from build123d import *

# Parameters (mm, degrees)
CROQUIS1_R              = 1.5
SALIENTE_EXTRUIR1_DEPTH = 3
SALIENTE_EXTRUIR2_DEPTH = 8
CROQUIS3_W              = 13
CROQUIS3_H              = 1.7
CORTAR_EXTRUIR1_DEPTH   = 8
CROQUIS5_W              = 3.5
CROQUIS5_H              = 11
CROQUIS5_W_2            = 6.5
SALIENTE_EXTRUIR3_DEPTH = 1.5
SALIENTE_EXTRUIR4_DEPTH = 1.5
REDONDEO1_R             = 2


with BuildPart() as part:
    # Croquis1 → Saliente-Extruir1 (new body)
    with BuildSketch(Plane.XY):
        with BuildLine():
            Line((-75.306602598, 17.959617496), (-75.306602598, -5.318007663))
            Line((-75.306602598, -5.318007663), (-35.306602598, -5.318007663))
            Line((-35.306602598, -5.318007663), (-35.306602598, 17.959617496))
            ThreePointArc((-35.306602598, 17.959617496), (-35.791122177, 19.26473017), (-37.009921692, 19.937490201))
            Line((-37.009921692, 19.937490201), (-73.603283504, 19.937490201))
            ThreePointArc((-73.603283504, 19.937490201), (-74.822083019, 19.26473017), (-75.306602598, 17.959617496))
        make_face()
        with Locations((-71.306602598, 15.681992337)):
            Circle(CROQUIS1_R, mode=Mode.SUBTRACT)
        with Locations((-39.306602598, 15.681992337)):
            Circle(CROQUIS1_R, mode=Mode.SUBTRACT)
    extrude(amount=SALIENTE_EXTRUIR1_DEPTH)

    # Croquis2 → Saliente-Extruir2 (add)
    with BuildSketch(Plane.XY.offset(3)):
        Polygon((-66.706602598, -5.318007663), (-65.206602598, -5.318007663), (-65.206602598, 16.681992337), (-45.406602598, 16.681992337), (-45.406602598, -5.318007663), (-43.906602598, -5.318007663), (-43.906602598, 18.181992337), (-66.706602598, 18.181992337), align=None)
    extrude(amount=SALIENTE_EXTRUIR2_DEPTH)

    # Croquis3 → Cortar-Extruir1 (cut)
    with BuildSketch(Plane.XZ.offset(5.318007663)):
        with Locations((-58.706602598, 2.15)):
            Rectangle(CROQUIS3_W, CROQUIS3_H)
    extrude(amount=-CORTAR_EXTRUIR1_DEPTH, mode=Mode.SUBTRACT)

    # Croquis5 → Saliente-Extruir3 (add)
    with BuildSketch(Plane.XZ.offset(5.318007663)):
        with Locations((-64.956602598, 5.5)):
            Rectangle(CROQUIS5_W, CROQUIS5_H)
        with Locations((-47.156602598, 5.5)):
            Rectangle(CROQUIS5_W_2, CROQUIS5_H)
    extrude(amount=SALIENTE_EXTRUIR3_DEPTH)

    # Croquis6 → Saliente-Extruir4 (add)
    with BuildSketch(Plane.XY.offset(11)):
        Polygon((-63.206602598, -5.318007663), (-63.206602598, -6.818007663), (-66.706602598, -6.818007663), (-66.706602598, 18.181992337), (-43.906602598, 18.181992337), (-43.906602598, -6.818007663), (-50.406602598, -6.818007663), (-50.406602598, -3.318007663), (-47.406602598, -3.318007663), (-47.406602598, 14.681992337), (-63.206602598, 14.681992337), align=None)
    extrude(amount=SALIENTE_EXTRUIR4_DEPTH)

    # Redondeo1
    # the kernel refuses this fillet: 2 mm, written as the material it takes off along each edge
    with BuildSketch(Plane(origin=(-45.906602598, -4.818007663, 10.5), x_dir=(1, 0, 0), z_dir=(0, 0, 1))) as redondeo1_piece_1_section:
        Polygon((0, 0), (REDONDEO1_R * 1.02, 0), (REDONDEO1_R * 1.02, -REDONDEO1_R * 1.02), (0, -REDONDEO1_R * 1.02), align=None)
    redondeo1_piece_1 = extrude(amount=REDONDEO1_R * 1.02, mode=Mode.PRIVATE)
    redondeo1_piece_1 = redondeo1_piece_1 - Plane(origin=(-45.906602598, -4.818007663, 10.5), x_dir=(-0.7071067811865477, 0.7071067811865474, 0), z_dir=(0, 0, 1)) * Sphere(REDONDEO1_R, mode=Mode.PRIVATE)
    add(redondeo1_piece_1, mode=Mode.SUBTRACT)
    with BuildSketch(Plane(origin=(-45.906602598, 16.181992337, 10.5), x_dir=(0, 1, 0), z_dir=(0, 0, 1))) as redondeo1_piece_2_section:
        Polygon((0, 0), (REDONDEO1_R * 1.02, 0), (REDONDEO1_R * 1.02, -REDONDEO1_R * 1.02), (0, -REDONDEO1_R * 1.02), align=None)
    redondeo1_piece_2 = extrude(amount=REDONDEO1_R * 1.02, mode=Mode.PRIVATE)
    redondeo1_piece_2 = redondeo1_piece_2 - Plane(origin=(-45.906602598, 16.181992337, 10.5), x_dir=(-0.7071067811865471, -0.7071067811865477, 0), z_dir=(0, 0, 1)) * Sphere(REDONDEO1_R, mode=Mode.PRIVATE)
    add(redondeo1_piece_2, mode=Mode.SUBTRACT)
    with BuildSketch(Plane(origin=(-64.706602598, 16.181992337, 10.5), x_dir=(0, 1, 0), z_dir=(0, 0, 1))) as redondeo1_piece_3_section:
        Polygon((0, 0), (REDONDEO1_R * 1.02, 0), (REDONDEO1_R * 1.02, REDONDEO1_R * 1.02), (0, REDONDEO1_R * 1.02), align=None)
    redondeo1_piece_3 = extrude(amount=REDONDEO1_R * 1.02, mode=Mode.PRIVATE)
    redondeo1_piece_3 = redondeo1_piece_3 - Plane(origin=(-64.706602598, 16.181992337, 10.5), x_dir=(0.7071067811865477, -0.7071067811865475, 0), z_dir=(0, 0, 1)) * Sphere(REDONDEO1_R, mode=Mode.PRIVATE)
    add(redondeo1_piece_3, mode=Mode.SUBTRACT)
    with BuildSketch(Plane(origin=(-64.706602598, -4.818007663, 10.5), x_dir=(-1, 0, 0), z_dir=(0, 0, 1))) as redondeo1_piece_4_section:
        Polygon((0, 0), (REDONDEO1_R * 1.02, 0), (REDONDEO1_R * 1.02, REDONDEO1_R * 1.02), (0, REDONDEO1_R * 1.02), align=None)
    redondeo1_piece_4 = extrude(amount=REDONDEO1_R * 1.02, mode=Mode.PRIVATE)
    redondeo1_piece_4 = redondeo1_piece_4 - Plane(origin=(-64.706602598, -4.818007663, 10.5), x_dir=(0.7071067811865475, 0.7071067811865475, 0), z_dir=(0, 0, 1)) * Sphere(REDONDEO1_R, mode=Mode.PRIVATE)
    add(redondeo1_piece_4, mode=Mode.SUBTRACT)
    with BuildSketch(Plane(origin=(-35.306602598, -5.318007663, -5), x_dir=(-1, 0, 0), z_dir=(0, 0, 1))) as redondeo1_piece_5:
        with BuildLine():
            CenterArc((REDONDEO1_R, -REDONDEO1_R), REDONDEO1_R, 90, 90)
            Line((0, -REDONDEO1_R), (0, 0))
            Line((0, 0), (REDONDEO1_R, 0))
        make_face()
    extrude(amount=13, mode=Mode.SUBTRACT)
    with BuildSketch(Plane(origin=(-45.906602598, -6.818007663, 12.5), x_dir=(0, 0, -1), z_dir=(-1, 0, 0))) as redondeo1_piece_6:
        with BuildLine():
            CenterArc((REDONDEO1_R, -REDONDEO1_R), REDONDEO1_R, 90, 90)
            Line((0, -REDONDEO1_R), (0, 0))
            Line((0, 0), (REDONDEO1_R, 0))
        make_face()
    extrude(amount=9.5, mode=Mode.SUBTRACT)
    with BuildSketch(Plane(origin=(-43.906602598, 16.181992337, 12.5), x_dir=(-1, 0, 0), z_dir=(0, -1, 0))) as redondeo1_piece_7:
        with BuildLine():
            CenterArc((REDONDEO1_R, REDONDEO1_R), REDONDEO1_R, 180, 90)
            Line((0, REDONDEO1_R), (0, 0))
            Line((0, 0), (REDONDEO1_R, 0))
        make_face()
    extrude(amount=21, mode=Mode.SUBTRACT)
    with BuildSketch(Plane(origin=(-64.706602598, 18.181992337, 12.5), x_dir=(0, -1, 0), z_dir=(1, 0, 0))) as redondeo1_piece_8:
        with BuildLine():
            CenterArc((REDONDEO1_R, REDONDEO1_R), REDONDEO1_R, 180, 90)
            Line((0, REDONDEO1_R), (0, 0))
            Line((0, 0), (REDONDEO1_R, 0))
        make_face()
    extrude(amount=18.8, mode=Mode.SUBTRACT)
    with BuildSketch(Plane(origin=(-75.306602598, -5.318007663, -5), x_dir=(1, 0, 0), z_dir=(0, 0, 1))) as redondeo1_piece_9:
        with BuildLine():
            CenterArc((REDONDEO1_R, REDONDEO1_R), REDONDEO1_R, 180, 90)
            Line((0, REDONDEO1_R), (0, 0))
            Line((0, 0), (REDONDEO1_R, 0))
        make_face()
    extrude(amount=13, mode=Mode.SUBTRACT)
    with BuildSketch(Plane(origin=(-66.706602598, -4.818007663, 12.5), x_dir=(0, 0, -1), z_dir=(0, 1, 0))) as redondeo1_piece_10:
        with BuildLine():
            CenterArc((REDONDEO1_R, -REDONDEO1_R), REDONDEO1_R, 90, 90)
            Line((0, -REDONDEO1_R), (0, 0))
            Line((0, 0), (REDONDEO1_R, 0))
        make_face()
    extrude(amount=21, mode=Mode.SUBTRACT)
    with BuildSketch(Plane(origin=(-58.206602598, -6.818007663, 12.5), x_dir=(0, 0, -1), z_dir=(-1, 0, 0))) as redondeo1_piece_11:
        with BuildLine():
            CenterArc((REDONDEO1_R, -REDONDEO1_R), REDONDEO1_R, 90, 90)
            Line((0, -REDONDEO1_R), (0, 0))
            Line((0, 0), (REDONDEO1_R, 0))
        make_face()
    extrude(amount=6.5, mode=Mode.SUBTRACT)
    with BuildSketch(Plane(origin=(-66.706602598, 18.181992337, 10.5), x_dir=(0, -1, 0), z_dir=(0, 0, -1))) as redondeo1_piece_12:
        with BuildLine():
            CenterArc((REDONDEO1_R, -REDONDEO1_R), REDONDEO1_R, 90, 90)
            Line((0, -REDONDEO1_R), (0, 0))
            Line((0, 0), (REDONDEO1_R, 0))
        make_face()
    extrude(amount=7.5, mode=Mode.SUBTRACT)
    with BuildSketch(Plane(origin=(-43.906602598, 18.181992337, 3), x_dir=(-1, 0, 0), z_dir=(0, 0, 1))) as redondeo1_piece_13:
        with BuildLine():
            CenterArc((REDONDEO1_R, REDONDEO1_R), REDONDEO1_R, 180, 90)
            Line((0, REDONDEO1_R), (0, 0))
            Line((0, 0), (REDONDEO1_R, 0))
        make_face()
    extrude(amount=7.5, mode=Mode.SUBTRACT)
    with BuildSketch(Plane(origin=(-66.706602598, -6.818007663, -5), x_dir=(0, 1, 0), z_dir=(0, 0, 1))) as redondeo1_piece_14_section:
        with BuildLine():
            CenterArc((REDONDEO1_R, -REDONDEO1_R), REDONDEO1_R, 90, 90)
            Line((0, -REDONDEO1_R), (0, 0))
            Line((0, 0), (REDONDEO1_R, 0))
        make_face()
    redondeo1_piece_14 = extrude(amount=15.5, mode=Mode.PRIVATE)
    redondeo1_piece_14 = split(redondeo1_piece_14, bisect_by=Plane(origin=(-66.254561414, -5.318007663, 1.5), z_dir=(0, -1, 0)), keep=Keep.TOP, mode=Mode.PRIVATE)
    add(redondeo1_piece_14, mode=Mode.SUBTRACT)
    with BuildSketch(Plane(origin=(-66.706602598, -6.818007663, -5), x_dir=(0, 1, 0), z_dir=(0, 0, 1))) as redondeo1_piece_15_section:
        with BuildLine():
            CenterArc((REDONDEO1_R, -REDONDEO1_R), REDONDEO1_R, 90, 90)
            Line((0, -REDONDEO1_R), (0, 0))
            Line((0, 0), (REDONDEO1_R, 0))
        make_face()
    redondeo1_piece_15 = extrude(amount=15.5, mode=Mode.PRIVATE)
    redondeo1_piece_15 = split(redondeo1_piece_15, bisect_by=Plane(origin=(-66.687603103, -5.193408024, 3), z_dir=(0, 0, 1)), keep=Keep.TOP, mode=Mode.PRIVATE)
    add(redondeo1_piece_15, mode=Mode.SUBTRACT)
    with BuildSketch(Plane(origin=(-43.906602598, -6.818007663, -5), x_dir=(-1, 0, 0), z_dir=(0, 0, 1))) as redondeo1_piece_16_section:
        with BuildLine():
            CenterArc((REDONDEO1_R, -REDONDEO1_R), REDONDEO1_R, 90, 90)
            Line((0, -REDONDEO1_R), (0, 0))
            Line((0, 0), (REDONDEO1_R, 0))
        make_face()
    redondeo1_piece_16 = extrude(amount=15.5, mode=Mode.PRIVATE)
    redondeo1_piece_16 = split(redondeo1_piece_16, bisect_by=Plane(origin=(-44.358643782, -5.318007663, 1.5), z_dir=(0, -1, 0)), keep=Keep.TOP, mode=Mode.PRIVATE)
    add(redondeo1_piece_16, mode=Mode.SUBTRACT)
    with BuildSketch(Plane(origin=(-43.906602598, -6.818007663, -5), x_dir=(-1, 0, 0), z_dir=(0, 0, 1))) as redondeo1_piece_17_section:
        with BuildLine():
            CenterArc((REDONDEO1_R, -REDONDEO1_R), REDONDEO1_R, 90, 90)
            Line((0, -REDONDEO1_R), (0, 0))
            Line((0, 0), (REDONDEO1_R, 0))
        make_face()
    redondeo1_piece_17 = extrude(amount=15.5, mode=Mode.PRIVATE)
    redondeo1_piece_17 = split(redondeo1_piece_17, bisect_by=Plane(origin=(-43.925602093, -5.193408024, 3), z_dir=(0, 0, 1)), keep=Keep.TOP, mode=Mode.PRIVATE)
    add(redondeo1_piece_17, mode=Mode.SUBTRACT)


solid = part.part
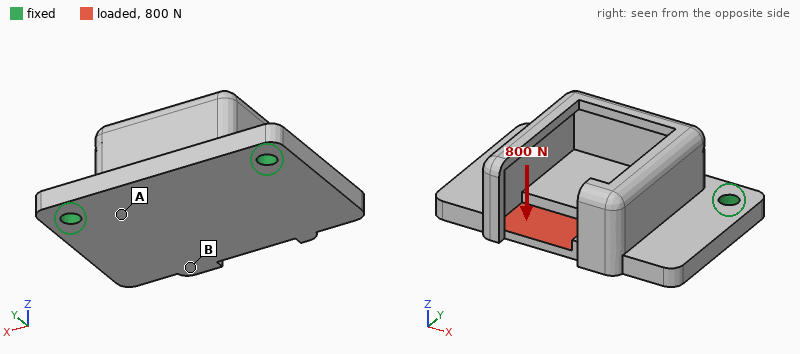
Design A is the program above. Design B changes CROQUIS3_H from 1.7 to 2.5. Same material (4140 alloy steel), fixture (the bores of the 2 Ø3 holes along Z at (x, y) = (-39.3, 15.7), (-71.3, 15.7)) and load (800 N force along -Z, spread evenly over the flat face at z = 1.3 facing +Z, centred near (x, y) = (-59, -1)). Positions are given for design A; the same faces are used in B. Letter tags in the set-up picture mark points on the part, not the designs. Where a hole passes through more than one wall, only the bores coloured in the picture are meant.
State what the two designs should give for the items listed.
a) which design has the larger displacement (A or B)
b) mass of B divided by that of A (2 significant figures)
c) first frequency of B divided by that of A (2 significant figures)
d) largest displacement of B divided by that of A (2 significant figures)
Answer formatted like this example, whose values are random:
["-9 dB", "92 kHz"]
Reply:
["B", "0.99", "1.0", "1.2"]
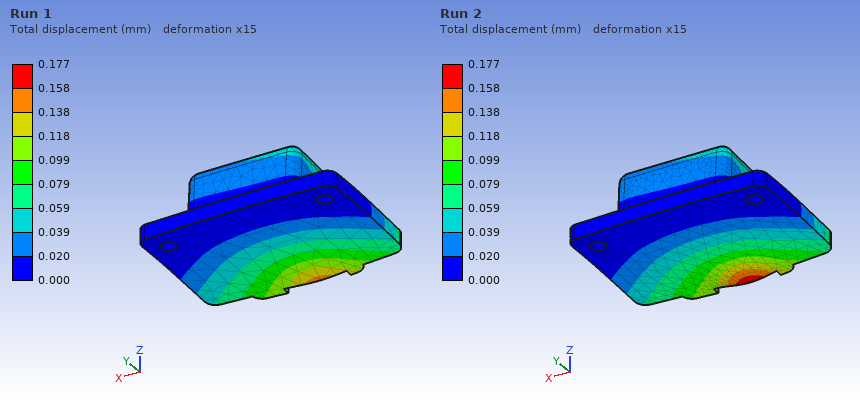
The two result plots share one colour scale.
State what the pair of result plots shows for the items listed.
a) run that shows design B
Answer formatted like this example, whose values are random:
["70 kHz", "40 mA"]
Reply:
["Run 2"]
